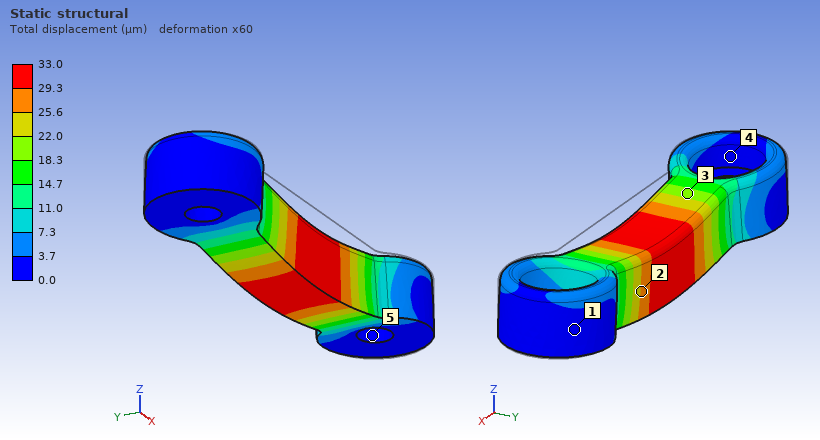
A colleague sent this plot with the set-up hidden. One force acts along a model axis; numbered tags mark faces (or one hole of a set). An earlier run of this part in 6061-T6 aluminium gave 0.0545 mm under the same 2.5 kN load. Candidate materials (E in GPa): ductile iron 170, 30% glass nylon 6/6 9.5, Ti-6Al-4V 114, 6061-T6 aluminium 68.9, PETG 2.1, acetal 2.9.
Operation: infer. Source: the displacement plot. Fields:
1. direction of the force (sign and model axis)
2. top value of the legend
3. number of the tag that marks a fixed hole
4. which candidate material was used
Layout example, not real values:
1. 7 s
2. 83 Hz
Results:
1. -Z
2. 33.0 µm
3. 5
4. Ti-6Al-4V
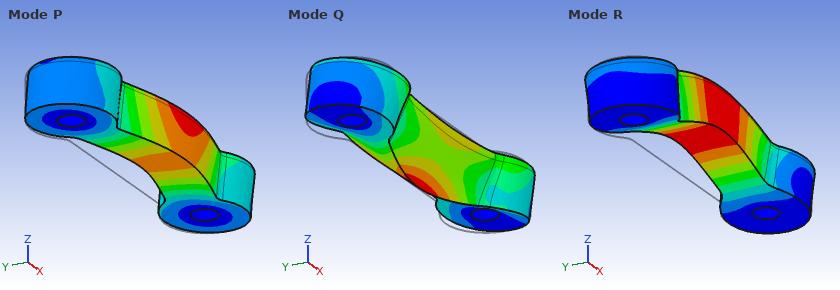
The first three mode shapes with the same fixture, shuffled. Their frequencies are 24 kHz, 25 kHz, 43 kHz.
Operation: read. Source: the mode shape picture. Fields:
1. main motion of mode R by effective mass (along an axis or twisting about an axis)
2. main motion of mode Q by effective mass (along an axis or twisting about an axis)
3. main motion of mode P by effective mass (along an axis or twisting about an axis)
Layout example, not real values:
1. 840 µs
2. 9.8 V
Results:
1. along Z
2. twisting about X
3. along Y
